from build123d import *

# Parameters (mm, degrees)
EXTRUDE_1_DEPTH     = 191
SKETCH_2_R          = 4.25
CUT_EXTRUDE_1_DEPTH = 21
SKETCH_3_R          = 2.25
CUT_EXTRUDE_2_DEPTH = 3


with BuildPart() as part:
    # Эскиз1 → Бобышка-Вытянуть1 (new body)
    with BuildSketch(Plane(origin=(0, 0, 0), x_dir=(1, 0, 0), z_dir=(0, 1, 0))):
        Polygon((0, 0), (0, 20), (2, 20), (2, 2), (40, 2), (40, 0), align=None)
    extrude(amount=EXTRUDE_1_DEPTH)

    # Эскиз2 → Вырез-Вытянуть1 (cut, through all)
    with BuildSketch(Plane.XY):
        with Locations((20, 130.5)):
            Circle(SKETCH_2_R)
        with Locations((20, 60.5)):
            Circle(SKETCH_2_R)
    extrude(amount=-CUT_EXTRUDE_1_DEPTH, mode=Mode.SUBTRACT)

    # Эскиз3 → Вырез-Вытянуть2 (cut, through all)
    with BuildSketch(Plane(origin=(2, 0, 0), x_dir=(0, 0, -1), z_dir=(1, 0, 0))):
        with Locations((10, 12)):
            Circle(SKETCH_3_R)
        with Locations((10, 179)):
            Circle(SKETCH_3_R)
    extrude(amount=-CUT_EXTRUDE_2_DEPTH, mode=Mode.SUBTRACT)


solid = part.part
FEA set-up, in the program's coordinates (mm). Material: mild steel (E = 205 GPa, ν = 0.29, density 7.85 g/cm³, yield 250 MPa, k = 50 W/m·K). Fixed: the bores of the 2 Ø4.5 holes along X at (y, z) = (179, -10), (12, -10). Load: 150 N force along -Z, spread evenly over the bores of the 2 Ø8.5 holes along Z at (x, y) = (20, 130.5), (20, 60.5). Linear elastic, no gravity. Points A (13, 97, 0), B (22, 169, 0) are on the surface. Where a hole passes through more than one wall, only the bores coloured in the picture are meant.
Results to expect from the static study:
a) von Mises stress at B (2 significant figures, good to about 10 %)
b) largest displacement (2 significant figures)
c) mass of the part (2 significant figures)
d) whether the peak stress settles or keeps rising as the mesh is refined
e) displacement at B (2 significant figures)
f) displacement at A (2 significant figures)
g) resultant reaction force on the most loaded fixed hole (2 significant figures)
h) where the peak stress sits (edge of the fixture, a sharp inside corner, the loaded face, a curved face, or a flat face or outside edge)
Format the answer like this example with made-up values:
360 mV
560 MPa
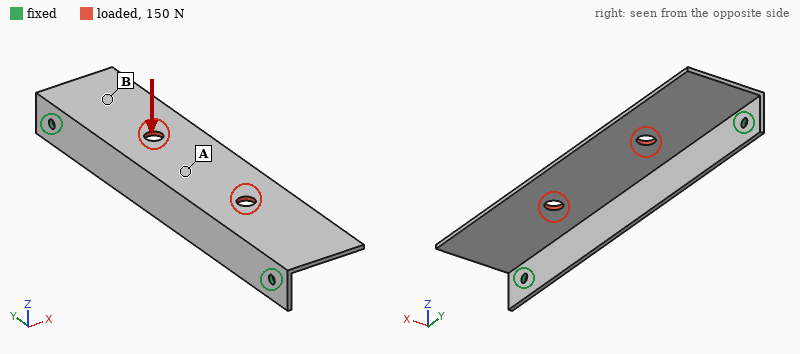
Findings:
19 MPa
0.30 mm
170 g
keeps rising
0.087 mm
0.10 mm
86 N
edge of the fixture
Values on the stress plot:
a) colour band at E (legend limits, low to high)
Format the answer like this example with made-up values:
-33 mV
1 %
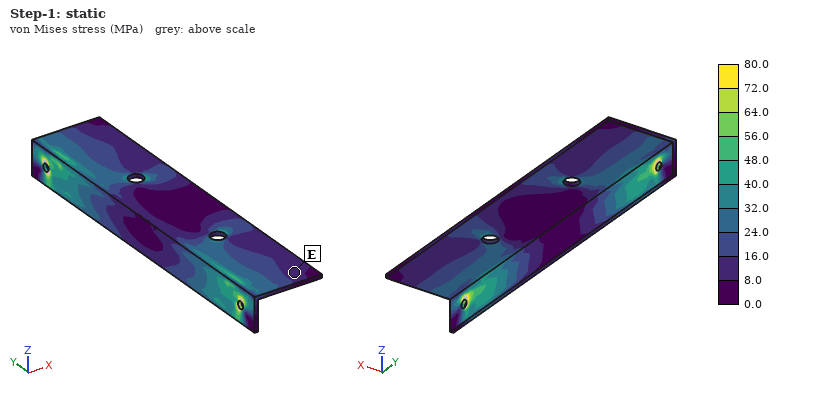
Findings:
8.0 to 16.0 MPa
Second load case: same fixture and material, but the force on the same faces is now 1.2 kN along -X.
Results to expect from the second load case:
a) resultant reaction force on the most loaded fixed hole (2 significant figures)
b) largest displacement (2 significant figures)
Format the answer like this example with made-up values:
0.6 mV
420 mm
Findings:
820 N
0.22 mm
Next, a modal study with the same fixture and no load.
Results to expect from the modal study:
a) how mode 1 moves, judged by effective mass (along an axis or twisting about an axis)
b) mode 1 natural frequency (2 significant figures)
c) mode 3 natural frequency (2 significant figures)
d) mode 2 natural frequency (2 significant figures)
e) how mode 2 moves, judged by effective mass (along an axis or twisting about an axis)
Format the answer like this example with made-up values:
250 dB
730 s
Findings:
along Z
450 Hz
1200 Hz
830 Hz
twisting about X
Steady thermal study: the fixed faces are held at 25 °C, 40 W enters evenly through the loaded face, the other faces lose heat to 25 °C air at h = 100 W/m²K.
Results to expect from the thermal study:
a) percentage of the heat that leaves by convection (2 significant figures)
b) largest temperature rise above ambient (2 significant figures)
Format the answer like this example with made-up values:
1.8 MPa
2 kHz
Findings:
95 %
69 K
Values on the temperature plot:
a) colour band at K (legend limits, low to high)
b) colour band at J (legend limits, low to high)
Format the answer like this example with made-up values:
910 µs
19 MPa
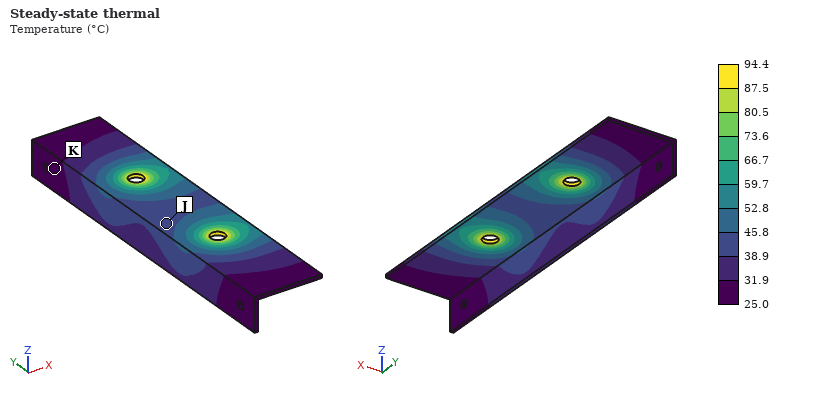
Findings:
25.0 to 31.9 °C
38.9 to 45.8 °C
